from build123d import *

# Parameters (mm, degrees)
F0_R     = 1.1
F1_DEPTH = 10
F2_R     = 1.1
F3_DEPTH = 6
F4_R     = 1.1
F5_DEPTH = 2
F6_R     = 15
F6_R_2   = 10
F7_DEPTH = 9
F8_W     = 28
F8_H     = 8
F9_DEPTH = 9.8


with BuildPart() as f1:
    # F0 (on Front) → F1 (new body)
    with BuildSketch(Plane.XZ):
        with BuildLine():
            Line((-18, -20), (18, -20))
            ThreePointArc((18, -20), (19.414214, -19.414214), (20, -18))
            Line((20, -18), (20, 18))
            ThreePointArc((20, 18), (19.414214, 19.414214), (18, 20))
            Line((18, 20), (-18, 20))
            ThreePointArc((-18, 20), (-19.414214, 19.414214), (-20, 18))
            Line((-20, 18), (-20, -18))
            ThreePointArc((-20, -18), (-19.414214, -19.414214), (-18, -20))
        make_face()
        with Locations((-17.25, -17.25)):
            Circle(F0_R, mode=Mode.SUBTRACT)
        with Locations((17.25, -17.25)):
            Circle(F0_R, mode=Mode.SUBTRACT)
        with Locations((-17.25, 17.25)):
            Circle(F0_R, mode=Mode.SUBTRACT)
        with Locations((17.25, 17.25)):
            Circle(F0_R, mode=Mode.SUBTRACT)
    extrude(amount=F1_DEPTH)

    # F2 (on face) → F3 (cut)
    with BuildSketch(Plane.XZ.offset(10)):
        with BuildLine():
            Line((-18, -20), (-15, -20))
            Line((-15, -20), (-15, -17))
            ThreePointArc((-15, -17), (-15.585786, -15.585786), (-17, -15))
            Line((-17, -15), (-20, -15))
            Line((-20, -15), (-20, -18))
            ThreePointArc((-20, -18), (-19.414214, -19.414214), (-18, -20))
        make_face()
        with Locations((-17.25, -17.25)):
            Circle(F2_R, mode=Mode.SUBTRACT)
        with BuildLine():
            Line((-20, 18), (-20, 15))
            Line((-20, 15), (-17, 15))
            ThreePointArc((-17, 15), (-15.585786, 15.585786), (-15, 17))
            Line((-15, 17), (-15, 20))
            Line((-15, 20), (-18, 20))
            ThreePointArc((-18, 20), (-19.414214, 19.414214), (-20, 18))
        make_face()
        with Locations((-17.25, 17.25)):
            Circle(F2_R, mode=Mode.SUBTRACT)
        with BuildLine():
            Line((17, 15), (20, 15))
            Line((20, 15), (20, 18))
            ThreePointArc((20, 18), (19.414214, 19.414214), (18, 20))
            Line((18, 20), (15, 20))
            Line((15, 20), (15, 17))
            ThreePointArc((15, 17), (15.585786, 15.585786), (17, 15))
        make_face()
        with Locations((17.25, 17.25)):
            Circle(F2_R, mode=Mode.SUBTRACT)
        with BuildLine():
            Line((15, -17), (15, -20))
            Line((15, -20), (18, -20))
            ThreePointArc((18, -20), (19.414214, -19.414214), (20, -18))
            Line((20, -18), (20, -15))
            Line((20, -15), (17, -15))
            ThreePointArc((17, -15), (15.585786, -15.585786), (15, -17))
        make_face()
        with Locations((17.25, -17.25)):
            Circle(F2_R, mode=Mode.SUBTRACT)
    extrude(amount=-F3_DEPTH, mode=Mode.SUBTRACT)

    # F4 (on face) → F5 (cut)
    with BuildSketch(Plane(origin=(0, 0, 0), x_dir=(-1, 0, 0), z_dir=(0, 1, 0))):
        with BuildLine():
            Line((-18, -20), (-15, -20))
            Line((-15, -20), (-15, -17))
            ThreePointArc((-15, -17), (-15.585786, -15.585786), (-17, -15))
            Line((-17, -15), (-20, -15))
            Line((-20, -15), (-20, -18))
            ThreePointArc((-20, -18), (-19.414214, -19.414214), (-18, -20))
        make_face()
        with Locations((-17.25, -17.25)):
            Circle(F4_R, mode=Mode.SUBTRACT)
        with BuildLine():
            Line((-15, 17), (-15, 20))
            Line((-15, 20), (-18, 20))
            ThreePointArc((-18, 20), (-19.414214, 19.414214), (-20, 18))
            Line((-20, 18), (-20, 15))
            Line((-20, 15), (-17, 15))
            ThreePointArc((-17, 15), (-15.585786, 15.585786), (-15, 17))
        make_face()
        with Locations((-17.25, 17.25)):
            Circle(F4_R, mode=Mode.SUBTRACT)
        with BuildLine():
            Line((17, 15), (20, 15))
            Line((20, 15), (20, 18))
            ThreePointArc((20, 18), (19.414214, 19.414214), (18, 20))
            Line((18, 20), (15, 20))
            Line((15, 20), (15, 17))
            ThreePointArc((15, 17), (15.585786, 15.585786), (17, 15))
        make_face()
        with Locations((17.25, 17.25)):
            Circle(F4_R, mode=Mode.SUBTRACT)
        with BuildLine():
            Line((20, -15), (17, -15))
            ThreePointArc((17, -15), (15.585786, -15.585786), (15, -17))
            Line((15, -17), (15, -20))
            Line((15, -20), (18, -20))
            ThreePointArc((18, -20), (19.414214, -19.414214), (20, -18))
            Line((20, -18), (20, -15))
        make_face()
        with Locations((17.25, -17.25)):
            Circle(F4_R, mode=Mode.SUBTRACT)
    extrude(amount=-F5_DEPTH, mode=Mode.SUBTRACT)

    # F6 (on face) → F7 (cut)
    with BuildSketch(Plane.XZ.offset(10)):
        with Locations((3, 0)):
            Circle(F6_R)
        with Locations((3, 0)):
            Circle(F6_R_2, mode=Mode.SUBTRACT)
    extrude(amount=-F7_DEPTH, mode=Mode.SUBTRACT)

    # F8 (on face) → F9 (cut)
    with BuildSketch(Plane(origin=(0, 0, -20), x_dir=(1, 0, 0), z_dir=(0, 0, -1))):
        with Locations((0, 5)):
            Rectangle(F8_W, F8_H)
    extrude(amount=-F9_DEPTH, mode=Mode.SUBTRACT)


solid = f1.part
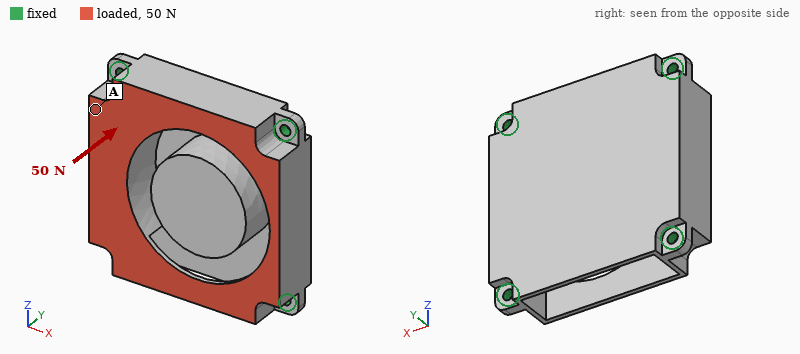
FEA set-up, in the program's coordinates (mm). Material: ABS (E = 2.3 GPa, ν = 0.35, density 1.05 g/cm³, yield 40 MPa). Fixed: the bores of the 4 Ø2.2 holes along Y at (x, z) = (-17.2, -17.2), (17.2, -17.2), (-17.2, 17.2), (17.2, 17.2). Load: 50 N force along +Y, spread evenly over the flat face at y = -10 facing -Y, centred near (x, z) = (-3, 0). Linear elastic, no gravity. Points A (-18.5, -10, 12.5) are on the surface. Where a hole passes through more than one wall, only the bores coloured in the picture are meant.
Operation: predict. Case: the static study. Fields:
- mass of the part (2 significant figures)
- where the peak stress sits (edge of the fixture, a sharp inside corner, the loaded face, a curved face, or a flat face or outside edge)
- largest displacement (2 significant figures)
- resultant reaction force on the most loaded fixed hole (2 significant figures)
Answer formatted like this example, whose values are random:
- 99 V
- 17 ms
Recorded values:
- 11 g
- the loaded face
- 0.49 mm
- 16 N
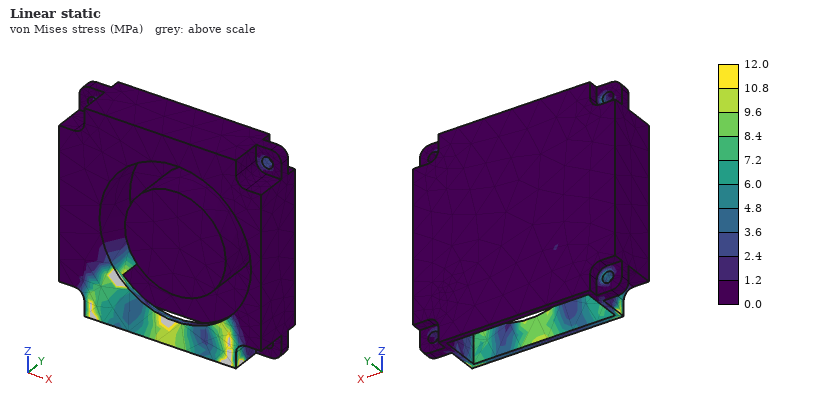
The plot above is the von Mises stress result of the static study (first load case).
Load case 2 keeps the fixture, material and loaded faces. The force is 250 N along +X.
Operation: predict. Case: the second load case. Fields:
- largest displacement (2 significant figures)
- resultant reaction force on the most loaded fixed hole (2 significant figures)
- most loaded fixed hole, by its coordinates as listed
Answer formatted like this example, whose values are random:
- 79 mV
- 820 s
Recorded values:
- 0.18 mm
- 83 N
- (17.2, 17.2)
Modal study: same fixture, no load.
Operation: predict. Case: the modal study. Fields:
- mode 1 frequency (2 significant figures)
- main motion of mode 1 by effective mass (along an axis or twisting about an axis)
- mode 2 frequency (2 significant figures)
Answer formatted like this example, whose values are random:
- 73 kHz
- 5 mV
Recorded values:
- 1800 Hz
- along Y
- 2200 Hz
